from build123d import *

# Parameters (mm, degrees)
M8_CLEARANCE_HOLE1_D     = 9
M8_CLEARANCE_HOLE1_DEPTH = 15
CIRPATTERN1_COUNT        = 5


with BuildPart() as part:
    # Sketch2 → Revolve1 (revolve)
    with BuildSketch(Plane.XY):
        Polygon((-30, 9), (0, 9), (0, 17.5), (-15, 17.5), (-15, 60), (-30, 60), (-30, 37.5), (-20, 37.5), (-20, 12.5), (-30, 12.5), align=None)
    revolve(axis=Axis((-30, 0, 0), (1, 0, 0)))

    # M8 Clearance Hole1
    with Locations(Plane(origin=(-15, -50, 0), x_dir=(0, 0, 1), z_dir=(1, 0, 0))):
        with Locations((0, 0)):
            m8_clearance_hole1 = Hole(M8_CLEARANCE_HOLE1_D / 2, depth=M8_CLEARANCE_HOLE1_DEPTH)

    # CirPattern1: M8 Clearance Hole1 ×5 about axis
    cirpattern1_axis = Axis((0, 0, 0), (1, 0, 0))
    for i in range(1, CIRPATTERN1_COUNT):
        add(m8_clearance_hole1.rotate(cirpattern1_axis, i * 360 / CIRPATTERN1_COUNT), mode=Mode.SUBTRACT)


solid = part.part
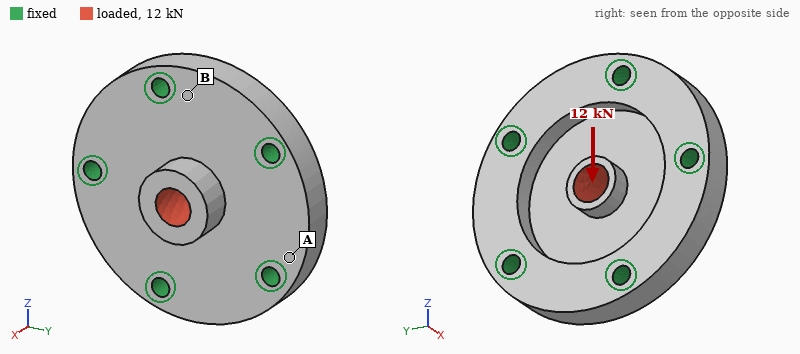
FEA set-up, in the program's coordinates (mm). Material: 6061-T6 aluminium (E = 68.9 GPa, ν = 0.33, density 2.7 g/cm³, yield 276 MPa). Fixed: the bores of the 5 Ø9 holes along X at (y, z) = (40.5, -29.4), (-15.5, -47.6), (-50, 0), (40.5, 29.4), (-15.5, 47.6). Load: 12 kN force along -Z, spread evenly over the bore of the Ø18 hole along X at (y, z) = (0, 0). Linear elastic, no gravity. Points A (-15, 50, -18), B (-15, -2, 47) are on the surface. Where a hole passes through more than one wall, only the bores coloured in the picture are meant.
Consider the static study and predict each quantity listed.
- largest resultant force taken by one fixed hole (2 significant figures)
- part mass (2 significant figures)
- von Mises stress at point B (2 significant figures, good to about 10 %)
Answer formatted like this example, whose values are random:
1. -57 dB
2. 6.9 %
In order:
1. 3.2 kN
2. 360 g
3. 9.7 MPa
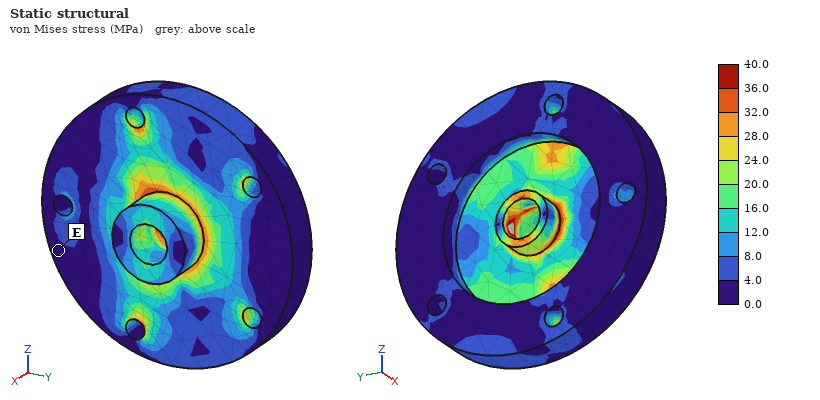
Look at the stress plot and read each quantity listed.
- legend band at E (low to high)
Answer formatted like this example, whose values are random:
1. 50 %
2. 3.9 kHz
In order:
1. 0.0 to 4.0 MPa
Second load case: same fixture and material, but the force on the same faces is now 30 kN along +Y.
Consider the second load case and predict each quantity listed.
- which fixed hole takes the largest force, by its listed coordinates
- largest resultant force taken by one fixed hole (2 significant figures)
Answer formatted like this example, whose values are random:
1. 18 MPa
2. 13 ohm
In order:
1. (-50, 0)
2. 8.4 kN
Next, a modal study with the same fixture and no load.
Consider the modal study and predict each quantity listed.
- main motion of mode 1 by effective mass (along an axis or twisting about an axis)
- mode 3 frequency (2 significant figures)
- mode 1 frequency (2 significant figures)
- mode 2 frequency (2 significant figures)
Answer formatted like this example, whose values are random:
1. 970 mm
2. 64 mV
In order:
1. along X
2. 9500 Hz
3. 6200 Hz
4. 9500 Hz
